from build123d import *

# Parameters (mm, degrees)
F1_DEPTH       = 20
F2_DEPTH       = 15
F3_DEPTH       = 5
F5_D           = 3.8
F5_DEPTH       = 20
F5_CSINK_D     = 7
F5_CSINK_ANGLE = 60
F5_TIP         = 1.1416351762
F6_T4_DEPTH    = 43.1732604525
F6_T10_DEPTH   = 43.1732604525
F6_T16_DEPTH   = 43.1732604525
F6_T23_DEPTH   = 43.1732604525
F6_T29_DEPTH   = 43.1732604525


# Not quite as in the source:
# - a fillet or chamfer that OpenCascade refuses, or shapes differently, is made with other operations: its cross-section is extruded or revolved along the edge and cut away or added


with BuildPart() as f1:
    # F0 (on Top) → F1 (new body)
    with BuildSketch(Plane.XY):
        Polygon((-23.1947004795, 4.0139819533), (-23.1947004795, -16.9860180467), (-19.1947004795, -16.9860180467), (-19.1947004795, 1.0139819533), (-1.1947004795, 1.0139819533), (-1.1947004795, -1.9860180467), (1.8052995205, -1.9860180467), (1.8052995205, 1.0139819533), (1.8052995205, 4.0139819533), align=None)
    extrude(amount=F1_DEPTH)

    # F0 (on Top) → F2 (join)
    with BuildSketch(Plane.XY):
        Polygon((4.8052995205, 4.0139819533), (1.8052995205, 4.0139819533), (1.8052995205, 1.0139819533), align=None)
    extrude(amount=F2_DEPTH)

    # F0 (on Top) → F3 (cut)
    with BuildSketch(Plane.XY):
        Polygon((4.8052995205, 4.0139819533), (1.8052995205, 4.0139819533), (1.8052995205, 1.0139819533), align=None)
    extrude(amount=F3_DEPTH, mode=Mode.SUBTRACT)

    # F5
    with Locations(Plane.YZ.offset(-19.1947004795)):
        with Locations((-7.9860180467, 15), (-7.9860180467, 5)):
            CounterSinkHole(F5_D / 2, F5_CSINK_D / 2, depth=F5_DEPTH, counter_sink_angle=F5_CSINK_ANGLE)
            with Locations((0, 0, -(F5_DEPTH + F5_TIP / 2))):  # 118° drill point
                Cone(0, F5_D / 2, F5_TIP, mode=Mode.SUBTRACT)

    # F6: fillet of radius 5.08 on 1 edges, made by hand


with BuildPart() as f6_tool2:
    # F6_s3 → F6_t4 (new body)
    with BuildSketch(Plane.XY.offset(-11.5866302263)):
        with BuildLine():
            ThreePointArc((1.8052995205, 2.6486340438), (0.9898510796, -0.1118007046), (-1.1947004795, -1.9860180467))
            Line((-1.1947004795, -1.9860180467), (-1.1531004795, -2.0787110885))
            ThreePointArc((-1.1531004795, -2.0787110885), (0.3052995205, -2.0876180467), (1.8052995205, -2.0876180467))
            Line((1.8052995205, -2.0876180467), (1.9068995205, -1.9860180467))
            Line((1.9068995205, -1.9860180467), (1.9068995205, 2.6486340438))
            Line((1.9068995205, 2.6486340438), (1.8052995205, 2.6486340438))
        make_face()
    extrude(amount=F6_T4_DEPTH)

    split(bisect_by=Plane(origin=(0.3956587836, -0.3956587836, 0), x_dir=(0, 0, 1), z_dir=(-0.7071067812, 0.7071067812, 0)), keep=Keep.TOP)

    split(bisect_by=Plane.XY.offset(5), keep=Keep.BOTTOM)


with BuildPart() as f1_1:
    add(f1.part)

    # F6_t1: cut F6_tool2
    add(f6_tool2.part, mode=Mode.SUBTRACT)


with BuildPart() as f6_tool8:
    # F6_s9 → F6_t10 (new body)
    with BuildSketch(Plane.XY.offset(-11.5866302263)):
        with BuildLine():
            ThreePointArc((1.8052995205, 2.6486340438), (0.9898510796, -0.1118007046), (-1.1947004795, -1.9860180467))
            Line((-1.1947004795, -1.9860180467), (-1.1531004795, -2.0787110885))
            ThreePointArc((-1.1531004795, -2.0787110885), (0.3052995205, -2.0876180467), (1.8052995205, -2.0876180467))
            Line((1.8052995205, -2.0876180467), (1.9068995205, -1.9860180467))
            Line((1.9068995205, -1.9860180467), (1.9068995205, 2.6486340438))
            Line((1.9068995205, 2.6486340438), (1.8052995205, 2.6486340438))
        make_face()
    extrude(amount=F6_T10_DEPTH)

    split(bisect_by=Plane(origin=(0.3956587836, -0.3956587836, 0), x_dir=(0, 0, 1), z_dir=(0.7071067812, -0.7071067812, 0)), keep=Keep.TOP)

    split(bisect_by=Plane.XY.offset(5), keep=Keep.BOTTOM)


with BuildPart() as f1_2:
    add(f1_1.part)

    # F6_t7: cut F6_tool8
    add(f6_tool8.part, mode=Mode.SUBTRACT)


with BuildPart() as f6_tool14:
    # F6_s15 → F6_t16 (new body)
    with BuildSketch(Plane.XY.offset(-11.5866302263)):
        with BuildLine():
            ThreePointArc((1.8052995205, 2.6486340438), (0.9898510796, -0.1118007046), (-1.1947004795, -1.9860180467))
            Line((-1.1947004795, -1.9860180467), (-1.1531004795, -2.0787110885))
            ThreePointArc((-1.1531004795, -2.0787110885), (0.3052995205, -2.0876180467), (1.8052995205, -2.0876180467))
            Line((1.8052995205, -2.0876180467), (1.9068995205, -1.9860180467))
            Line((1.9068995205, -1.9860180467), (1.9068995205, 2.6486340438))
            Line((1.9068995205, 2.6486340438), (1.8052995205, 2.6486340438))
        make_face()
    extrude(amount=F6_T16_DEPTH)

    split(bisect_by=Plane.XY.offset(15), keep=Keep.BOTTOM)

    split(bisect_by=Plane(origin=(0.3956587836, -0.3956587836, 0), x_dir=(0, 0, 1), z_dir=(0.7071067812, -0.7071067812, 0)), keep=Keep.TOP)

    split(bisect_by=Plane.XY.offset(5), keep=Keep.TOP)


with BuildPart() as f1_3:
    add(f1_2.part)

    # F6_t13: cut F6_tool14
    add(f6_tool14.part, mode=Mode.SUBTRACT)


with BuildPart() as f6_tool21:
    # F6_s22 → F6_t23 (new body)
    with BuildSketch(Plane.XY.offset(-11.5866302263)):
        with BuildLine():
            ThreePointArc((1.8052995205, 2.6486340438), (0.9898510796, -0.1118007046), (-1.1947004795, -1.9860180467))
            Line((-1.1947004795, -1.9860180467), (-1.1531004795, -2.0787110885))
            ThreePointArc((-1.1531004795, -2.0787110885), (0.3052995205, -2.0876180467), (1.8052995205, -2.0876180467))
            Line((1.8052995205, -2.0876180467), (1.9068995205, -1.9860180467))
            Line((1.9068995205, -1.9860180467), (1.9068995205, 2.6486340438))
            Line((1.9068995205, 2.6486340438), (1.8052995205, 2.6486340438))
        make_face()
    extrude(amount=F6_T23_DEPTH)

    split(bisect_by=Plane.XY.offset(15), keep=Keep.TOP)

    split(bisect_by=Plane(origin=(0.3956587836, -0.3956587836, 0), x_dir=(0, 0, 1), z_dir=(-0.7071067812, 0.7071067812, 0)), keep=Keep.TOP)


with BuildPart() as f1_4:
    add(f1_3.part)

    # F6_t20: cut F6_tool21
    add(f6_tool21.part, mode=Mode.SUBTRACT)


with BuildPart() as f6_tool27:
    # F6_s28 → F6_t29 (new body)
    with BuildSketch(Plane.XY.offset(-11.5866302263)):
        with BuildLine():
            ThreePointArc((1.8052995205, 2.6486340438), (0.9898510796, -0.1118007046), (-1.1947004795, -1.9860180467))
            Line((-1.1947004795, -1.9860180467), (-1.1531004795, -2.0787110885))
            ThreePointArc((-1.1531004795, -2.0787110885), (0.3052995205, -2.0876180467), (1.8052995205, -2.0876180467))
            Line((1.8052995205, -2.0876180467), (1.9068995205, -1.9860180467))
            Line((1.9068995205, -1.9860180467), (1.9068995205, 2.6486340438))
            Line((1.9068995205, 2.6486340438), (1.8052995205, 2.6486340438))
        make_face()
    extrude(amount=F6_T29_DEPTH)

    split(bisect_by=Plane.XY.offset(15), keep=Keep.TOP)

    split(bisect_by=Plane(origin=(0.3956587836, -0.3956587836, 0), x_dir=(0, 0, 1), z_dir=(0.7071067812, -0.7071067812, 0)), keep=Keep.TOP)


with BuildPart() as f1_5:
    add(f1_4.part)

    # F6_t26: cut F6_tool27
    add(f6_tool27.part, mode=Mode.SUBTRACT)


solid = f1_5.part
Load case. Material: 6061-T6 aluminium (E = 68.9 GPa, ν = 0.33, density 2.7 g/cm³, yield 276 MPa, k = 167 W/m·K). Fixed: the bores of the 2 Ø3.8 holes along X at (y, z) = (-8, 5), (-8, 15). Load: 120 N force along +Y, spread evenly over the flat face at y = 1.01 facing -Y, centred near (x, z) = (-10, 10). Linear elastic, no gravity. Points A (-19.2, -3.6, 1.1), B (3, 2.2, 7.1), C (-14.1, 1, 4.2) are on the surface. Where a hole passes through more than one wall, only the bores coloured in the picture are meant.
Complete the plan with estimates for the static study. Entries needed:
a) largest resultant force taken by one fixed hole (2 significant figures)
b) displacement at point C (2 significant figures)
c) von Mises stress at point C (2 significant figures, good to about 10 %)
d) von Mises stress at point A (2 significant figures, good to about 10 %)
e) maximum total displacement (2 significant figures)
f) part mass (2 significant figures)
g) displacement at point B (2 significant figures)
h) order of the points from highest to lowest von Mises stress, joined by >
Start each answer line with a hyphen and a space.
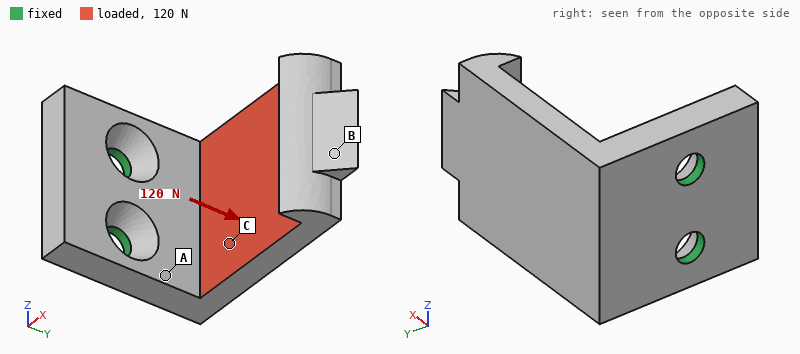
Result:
- 61 N
- 0.032 mm
- 17 MPa
- 32 MPa
- 0.13 mm
- 7.9 g
- 0.12 mm
- A > C > B
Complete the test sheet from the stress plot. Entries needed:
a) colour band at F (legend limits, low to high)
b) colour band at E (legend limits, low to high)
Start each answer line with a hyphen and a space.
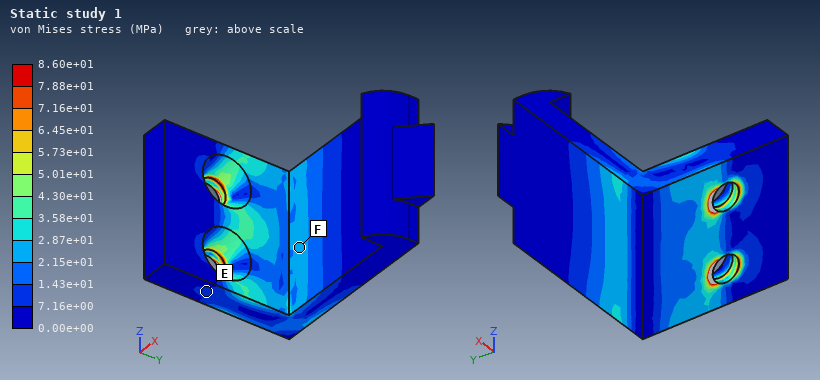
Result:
- 2.15e+01 to 2.87e+01 MPa
- 7.16e+00 to 1.43e+01 MPa
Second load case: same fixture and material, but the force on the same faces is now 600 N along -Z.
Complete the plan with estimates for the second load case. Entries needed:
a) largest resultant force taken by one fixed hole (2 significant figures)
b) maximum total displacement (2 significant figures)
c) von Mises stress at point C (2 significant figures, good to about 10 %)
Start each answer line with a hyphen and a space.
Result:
- 870 N
- 0.15 mm
- 48 MPa
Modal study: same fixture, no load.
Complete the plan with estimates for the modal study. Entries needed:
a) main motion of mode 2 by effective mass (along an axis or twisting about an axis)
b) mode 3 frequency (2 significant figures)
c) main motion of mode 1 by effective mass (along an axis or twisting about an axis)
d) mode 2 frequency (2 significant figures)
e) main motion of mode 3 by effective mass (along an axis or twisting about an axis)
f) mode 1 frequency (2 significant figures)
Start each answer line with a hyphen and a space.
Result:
- along Z
- 8800 Hz
- along Y
- 5500 Hz
- along X
- 2700 Hz
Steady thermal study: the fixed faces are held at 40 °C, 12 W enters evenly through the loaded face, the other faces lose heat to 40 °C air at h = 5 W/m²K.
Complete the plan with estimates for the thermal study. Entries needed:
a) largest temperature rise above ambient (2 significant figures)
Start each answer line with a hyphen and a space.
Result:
- 22 K
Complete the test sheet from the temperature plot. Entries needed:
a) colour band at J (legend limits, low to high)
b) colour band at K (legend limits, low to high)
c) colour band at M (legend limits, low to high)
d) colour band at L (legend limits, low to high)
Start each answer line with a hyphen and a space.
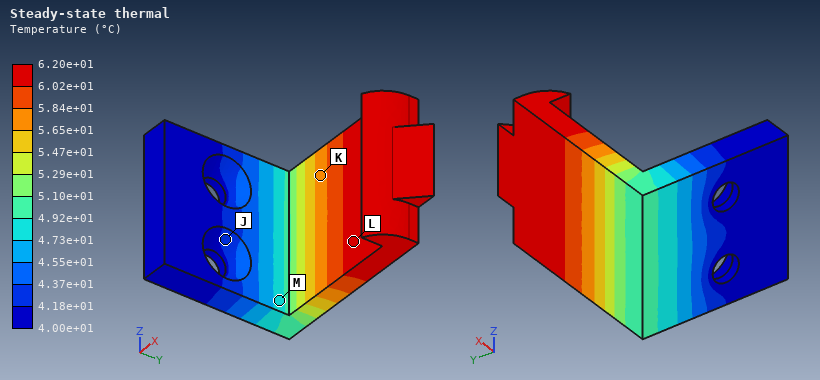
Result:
- 4.18e+01 to 4.37e+01 °C
- 5.65e+01 to 5.84e+01 °C
- 4.73e+01 to 4.92e+01 °C
- 6.02e+01 to 6.20e+01 °C
